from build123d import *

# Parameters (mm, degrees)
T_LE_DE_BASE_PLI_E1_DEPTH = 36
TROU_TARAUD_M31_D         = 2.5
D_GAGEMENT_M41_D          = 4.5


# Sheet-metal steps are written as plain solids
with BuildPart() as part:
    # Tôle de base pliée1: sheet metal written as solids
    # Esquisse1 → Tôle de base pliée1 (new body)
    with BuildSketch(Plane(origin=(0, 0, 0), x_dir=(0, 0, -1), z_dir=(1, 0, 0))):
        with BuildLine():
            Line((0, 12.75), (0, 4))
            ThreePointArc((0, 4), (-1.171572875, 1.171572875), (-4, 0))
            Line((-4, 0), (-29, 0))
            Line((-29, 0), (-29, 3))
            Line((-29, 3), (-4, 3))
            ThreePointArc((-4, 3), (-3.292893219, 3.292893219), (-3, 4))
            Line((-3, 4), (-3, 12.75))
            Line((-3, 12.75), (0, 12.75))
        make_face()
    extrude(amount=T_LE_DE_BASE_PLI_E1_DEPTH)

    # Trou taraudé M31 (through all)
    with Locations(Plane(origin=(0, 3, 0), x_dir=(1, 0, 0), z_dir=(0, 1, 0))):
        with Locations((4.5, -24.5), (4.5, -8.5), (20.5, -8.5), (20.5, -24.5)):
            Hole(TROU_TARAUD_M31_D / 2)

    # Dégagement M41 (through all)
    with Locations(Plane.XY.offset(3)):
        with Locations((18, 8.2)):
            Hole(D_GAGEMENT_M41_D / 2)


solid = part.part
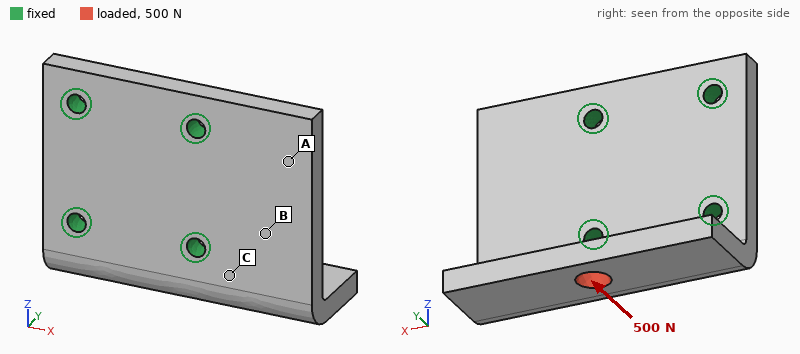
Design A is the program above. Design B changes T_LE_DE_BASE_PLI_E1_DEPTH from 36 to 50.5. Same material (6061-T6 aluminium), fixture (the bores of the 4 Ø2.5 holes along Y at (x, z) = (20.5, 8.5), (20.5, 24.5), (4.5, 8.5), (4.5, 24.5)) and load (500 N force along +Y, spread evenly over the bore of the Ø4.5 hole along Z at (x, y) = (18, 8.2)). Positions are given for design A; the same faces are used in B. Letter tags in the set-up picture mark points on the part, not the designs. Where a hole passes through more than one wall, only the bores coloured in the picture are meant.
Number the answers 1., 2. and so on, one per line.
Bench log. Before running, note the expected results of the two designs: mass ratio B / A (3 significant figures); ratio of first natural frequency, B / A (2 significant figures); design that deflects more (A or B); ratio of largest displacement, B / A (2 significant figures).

1. 1.41
2. 0.45
3. A
4. 0.92
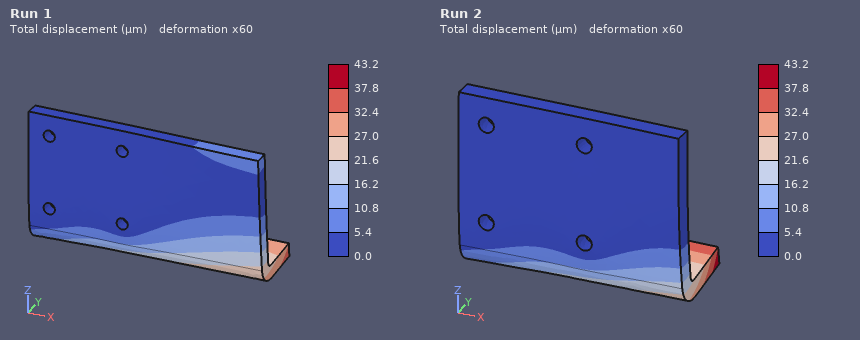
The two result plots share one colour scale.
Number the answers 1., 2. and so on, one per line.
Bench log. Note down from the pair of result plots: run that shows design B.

1. Run 1
